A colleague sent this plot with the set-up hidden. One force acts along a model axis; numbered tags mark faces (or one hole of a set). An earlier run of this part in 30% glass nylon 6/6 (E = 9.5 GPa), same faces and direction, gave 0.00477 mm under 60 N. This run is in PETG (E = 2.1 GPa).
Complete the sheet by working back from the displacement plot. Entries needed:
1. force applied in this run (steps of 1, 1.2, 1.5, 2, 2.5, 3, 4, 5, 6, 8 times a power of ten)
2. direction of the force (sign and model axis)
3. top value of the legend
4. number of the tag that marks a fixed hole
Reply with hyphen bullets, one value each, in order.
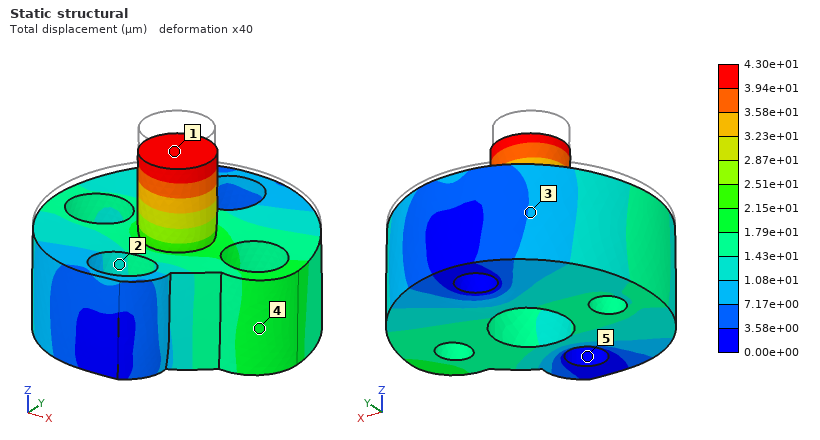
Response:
- 120 N
- -Z
- 4.30e+01 µm
- 5
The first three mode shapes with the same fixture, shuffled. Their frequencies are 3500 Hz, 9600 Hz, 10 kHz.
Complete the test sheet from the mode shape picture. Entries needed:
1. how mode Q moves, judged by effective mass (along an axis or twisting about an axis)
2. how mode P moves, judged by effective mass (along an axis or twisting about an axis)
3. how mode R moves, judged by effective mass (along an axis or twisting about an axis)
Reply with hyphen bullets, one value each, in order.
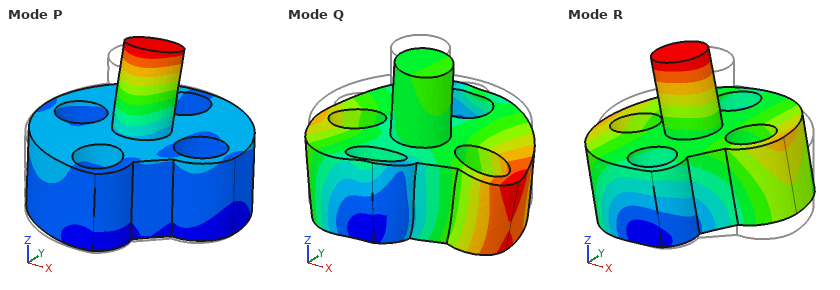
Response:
- along Z
- along Y
- along X
